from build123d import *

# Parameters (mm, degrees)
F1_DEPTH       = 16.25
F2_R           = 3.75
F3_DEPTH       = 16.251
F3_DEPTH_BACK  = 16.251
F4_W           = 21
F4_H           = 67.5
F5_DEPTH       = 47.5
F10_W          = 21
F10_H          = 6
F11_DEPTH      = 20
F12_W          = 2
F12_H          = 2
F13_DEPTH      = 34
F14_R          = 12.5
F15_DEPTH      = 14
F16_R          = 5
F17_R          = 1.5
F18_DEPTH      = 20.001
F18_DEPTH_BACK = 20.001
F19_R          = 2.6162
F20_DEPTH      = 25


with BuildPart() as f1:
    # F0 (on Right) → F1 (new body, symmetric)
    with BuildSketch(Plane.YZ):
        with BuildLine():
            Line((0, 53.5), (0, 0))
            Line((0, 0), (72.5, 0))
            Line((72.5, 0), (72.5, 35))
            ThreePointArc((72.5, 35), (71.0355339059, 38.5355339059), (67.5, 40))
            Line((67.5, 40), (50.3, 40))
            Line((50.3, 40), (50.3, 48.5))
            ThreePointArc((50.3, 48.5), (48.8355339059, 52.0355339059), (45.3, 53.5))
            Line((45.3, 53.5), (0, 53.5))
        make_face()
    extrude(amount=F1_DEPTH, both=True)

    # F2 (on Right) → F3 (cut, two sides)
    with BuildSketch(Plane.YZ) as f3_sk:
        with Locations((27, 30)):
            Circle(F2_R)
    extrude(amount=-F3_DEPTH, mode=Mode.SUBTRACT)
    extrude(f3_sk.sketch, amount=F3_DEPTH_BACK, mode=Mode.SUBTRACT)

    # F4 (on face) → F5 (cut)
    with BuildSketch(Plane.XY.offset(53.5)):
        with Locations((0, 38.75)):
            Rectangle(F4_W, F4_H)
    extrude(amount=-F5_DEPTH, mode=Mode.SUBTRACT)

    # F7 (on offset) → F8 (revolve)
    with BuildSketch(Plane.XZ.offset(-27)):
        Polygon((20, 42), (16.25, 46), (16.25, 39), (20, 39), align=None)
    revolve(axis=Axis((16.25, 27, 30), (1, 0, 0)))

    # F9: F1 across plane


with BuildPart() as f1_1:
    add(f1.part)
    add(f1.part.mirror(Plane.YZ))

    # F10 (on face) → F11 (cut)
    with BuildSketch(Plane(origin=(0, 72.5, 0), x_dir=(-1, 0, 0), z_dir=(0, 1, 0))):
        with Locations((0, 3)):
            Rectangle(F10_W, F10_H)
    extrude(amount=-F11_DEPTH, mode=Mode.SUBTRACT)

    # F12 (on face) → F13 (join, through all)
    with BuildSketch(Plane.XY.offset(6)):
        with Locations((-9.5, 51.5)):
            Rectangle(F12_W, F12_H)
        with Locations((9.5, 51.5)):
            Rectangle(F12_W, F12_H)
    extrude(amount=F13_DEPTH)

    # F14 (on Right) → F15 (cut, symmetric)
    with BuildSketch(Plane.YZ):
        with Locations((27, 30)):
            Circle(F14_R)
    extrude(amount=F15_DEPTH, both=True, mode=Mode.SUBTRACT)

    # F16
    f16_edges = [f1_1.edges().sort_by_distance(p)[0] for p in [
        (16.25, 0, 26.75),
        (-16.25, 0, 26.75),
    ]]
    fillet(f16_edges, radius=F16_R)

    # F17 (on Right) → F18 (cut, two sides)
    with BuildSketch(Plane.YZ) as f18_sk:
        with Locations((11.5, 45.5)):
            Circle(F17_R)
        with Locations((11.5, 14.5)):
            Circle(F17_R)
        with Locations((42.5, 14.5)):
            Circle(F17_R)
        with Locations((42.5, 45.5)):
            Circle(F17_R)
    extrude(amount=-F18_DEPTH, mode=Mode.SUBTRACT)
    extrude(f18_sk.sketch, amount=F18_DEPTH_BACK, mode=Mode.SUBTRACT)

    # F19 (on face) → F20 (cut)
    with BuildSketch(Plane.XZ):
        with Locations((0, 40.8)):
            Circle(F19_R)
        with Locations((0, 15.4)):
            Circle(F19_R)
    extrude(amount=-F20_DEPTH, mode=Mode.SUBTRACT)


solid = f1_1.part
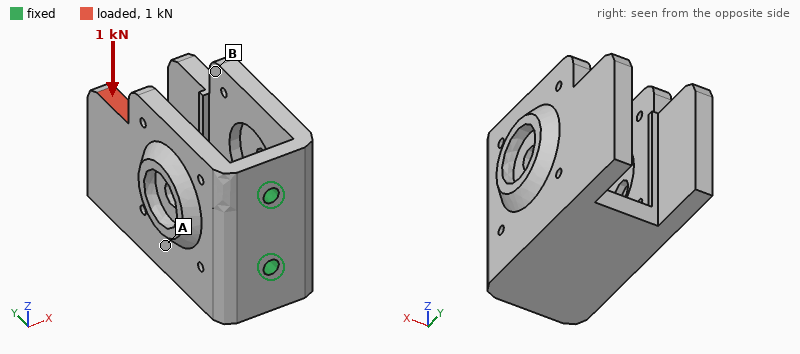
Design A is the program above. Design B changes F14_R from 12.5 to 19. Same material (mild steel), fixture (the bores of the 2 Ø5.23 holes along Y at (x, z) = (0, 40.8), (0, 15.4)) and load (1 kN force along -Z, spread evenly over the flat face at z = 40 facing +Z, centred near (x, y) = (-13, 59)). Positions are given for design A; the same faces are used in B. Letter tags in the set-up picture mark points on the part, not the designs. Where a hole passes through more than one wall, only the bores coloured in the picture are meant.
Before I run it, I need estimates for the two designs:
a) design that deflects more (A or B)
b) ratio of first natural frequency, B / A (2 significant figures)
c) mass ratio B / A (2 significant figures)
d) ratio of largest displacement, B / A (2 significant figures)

B
0.99
0.91
1.2
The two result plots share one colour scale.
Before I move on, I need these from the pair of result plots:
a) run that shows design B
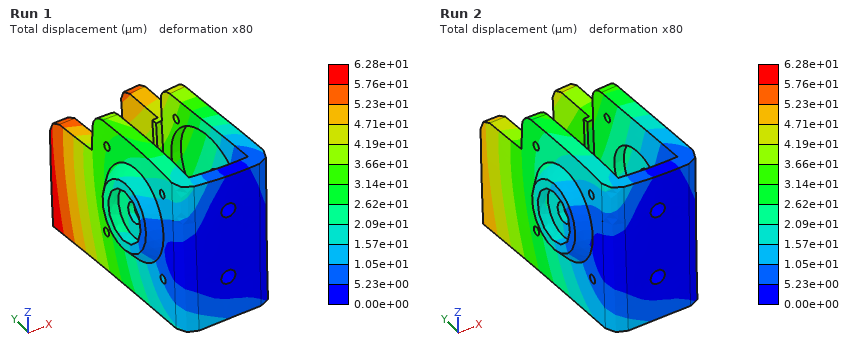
Run 1
